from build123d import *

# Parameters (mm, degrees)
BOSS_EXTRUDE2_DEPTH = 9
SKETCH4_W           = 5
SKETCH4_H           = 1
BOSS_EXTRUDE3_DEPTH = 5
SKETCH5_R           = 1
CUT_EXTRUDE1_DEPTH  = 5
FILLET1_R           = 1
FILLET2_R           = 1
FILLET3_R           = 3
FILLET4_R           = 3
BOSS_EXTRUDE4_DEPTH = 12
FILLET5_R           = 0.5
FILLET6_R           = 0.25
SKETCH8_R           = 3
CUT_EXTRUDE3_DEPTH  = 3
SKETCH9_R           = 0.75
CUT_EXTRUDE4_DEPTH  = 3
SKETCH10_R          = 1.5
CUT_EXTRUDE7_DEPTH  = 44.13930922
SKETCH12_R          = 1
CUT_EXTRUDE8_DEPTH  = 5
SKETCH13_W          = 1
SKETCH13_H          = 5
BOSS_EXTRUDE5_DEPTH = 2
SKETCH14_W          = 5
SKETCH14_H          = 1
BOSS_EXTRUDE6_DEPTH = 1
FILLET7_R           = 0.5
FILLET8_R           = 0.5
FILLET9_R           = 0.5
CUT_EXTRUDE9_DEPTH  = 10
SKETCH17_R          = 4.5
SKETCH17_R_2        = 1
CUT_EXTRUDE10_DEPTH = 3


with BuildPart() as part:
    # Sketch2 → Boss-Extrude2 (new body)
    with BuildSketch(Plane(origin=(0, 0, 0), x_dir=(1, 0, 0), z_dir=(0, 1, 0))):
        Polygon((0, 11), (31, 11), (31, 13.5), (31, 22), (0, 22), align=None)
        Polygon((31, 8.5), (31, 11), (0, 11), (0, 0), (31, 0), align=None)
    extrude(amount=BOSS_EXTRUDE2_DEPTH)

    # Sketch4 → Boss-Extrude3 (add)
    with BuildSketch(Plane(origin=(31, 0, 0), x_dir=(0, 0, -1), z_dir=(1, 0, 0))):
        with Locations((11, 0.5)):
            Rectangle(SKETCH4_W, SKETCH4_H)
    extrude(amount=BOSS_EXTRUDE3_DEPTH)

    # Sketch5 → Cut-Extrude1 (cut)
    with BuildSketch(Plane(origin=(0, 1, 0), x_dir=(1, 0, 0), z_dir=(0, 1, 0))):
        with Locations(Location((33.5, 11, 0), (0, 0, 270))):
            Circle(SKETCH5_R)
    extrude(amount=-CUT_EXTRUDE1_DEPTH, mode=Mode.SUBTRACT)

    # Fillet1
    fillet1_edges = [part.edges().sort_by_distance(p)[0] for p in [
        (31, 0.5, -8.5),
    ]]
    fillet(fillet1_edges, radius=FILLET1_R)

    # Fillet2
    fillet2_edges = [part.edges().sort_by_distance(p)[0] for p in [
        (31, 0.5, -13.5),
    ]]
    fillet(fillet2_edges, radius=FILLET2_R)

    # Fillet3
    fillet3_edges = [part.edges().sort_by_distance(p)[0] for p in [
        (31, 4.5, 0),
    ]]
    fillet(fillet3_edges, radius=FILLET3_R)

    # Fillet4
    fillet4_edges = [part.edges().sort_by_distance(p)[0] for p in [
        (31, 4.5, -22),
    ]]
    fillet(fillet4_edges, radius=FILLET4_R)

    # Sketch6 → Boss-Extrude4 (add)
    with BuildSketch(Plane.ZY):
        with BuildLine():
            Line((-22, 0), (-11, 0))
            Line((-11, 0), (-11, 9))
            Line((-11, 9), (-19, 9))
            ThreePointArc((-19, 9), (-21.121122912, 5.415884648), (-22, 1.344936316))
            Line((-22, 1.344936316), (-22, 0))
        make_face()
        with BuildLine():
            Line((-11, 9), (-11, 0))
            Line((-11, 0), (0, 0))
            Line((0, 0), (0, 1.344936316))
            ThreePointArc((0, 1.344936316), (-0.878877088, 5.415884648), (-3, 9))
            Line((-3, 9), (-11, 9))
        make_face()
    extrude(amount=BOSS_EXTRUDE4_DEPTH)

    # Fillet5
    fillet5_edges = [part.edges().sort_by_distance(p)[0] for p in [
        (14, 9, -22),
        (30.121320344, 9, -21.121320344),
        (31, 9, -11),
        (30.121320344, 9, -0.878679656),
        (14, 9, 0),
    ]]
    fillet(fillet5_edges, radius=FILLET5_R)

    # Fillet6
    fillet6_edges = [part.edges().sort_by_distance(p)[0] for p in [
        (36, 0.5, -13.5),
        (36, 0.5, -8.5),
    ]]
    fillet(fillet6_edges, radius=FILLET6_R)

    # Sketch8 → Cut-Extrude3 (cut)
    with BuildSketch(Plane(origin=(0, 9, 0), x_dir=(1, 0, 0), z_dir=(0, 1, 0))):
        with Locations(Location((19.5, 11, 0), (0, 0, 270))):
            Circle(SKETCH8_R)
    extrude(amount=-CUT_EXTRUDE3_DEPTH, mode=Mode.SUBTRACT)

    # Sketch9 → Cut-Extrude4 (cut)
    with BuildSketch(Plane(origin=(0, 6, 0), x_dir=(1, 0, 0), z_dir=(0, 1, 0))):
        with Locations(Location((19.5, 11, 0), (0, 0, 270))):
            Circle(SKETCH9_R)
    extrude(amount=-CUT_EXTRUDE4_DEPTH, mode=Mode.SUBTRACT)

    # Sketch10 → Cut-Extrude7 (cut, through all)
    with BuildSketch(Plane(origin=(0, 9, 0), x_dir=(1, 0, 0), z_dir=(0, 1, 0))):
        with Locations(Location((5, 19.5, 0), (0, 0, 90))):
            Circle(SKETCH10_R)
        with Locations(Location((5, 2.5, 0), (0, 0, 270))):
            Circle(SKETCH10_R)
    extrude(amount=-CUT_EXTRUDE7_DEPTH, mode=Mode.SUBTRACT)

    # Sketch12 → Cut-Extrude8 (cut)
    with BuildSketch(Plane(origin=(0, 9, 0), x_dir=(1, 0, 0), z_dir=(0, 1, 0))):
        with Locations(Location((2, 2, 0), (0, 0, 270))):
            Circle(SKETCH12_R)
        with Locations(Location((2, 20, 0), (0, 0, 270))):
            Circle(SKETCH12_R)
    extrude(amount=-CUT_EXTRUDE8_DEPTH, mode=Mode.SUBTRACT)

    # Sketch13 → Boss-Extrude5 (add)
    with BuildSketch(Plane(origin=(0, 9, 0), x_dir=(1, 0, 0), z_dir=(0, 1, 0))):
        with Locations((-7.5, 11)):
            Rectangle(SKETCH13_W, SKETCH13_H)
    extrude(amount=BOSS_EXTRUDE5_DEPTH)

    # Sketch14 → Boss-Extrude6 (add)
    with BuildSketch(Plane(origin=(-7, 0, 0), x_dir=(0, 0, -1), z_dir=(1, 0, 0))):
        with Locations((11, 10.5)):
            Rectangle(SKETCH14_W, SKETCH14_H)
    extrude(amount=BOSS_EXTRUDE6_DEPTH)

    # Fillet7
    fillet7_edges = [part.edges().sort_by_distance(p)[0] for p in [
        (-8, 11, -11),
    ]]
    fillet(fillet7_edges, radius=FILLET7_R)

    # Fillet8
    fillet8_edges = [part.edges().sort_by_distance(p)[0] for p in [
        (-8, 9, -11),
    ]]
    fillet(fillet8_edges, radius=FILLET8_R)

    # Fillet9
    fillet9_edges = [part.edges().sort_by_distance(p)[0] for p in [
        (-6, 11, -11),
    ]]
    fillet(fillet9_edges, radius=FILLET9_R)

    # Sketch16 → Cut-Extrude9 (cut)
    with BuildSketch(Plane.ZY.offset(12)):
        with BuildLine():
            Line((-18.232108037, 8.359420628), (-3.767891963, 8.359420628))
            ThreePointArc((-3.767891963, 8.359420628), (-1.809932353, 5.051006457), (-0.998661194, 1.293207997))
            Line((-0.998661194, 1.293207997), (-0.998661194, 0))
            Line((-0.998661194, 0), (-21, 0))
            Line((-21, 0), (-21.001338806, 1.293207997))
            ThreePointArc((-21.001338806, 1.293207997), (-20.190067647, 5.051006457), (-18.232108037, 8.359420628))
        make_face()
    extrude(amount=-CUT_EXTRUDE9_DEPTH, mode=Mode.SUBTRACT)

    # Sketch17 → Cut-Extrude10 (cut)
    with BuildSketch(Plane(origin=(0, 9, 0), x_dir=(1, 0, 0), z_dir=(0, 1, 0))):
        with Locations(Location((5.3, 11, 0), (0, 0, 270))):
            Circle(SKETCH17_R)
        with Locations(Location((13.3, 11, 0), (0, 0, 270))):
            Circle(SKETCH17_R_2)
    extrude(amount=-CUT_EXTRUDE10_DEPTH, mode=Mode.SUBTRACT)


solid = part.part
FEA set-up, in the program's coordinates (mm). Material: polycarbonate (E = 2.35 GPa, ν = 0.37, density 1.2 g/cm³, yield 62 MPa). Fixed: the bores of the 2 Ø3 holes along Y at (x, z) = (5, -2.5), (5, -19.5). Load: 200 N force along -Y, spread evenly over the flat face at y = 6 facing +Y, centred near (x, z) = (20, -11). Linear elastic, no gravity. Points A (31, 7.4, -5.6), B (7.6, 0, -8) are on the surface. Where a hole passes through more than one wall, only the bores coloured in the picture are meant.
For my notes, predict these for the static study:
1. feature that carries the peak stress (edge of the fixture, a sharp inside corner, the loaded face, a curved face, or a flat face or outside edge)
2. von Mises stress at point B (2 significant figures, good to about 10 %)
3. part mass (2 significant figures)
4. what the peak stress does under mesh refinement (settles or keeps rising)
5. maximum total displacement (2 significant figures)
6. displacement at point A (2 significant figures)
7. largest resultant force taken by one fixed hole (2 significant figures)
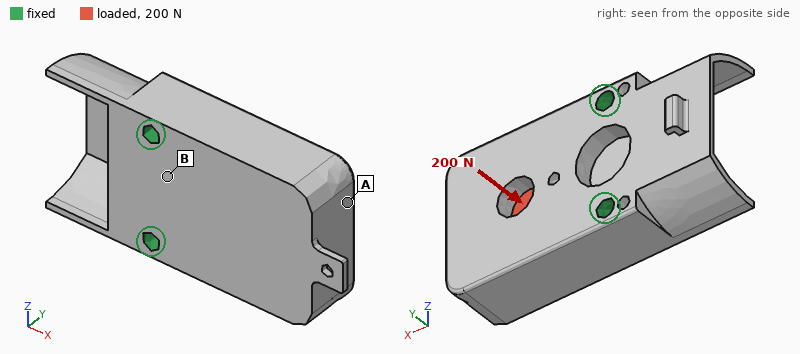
edge of the fixture
5.0 MPa
7.6 g
keeps rising
0.25 mm
0.20 mm
100 N
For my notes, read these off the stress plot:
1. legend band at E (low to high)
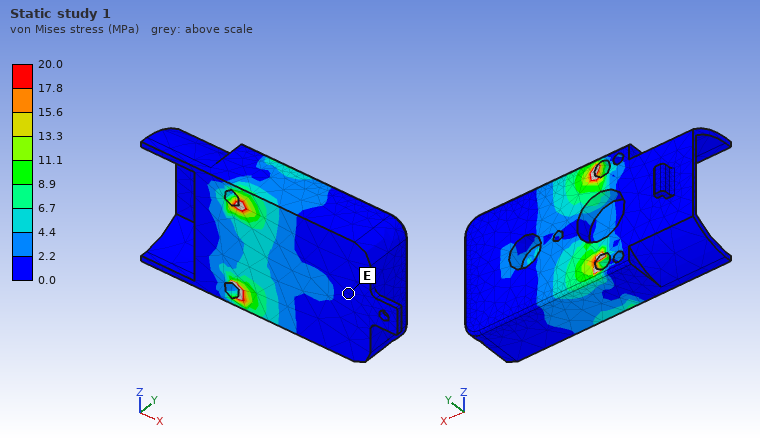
0.0 to 2.2 MPa
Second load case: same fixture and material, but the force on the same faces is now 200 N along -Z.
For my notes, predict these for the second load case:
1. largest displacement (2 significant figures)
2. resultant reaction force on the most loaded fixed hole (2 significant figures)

51 µm
180 N
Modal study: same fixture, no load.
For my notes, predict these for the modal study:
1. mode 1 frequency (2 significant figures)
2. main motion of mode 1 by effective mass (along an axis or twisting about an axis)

2500 Hz
along Y
